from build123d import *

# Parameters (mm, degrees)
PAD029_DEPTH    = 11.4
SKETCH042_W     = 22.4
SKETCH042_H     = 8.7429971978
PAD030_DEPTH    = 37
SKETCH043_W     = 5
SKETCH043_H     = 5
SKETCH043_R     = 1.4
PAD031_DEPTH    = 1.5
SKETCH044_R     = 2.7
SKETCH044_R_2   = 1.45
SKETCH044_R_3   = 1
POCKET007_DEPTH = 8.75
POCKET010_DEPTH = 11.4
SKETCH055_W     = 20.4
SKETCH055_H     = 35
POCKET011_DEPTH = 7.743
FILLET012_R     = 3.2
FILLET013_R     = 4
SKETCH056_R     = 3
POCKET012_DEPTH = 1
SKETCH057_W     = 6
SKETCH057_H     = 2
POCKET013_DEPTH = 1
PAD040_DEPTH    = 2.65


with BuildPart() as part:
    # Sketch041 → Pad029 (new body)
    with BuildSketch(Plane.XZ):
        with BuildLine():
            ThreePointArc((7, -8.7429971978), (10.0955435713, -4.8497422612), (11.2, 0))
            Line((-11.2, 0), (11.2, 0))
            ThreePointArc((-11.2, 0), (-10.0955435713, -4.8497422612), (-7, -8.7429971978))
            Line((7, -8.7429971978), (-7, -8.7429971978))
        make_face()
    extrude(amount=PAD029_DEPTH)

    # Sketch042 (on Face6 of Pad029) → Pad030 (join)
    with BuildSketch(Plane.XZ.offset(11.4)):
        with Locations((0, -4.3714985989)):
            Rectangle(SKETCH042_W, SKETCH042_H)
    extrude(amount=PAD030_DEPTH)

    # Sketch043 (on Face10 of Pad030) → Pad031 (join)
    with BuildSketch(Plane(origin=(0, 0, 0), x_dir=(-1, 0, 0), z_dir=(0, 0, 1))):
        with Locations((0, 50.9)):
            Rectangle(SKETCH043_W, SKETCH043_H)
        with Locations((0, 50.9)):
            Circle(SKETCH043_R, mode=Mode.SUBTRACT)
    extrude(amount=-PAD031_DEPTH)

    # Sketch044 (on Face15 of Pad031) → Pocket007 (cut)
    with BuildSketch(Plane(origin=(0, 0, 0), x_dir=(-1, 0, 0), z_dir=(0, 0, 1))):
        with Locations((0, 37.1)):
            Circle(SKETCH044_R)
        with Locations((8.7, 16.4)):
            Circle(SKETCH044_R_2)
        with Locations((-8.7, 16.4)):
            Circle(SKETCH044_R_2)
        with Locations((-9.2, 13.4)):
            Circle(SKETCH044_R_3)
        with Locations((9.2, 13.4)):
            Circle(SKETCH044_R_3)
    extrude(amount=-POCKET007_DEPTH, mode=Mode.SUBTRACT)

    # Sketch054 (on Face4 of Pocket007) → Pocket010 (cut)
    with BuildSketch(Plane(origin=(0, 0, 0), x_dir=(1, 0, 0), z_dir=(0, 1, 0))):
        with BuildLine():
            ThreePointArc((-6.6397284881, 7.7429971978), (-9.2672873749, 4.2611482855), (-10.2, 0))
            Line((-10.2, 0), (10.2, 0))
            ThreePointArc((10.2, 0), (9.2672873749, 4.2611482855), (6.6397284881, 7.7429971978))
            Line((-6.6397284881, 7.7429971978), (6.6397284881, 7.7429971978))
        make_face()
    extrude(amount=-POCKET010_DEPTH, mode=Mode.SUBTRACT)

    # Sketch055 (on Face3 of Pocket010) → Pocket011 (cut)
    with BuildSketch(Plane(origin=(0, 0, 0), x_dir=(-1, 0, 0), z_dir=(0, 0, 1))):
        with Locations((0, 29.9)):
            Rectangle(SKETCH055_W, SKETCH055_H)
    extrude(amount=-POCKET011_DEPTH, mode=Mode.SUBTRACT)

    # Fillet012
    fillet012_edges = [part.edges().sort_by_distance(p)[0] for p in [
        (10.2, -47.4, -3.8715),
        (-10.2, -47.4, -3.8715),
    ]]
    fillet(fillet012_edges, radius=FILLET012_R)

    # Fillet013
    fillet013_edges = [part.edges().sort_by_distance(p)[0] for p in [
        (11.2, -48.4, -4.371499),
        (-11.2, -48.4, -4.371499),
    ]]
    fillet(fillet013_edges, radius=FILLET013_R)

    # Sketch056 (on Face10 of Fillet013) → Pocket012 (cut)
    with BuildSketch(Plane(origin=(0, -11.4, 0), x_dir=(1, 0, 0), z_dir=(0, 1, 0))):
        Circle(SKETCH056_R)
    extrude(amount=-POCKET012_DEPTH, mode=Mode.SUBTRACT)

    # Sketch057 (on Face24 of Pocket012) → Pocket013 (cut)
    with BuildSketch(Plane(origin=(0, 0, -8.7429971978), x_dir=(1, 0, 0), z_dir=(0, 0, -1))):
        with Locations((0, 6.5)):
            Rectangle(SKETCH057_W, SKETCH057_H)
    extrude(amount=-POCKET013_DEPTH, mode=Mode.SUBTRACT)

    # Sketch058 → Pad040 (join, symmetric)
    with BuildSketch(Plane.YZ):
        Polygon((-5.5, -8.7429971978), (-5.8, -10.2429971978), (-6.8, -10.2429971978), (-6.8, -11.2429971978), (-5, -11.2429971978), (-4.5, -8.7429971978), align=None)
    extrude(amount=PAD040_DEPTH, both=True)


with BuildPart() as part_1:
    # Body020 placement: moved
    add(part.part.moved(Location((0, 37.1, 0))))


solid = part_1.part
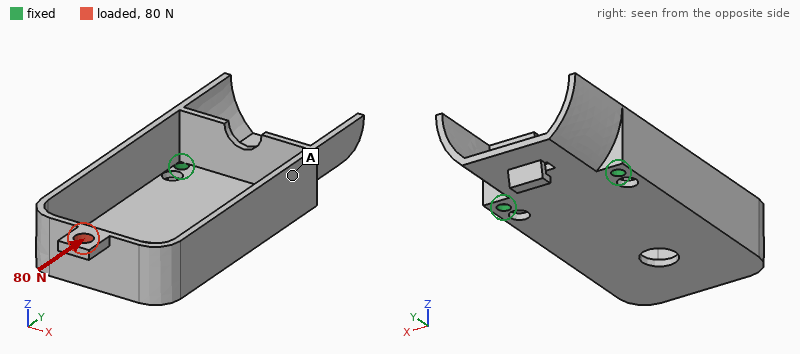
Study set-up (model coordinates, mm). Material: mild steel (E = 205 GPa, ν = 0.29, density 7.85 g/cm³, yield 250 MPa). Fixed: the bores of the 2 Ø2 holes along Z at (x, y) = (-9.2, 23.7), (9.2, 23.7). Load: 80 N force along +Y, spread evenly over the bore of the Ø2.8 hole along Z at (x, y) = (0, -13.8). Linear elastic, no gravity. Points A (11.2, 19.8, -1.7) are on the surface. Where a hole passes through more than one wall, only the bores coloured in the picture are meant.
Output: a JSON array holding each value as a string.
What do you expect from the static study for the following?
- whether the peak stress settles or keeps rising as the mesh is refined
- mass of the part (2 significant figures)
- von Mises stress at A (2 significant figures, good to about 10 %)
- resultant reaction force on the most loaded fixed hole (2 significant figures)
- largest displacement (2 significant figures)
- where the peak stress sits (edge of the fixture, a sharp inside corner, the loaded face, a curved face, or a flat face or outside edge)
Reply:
["keeps rising", "16 g", "14 MPa", "40 N", "82 µm", "edge of the fixture"]
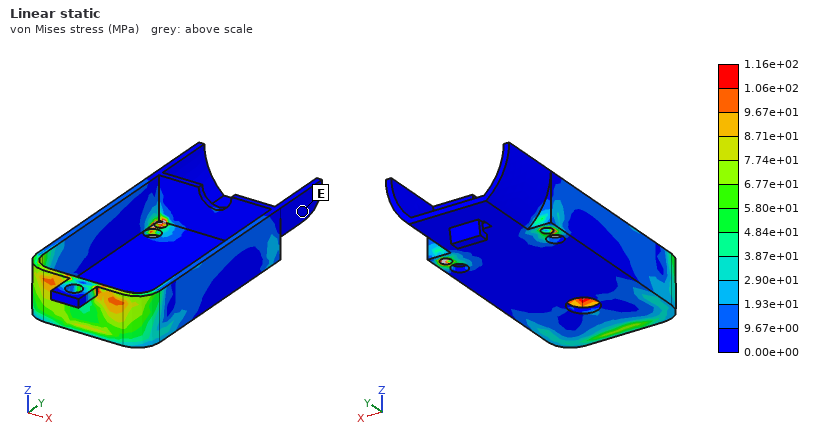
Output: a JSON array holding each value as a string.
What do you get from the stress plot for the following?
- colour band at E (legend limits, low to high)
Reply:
["0.00e+00 to 9.67e+00 MPa"]
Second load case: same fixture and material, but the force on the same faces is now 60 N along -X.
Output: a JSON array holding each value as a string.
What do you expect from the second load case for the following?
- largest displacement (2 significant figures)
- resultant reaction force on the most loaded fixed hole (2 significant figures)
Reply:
["63 µm", "120 N"]
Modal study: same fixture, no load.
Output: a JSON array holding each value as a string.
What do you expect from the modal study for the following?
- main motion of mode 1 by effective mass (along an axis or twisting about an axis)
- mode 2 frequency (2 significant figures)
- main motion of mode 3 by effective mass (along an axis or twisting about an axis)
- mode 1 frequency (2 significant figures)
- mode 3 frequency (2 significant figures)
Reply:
["along Z", "2600 Hz", "along X", "1600 Hz", "7600 Hz"]
